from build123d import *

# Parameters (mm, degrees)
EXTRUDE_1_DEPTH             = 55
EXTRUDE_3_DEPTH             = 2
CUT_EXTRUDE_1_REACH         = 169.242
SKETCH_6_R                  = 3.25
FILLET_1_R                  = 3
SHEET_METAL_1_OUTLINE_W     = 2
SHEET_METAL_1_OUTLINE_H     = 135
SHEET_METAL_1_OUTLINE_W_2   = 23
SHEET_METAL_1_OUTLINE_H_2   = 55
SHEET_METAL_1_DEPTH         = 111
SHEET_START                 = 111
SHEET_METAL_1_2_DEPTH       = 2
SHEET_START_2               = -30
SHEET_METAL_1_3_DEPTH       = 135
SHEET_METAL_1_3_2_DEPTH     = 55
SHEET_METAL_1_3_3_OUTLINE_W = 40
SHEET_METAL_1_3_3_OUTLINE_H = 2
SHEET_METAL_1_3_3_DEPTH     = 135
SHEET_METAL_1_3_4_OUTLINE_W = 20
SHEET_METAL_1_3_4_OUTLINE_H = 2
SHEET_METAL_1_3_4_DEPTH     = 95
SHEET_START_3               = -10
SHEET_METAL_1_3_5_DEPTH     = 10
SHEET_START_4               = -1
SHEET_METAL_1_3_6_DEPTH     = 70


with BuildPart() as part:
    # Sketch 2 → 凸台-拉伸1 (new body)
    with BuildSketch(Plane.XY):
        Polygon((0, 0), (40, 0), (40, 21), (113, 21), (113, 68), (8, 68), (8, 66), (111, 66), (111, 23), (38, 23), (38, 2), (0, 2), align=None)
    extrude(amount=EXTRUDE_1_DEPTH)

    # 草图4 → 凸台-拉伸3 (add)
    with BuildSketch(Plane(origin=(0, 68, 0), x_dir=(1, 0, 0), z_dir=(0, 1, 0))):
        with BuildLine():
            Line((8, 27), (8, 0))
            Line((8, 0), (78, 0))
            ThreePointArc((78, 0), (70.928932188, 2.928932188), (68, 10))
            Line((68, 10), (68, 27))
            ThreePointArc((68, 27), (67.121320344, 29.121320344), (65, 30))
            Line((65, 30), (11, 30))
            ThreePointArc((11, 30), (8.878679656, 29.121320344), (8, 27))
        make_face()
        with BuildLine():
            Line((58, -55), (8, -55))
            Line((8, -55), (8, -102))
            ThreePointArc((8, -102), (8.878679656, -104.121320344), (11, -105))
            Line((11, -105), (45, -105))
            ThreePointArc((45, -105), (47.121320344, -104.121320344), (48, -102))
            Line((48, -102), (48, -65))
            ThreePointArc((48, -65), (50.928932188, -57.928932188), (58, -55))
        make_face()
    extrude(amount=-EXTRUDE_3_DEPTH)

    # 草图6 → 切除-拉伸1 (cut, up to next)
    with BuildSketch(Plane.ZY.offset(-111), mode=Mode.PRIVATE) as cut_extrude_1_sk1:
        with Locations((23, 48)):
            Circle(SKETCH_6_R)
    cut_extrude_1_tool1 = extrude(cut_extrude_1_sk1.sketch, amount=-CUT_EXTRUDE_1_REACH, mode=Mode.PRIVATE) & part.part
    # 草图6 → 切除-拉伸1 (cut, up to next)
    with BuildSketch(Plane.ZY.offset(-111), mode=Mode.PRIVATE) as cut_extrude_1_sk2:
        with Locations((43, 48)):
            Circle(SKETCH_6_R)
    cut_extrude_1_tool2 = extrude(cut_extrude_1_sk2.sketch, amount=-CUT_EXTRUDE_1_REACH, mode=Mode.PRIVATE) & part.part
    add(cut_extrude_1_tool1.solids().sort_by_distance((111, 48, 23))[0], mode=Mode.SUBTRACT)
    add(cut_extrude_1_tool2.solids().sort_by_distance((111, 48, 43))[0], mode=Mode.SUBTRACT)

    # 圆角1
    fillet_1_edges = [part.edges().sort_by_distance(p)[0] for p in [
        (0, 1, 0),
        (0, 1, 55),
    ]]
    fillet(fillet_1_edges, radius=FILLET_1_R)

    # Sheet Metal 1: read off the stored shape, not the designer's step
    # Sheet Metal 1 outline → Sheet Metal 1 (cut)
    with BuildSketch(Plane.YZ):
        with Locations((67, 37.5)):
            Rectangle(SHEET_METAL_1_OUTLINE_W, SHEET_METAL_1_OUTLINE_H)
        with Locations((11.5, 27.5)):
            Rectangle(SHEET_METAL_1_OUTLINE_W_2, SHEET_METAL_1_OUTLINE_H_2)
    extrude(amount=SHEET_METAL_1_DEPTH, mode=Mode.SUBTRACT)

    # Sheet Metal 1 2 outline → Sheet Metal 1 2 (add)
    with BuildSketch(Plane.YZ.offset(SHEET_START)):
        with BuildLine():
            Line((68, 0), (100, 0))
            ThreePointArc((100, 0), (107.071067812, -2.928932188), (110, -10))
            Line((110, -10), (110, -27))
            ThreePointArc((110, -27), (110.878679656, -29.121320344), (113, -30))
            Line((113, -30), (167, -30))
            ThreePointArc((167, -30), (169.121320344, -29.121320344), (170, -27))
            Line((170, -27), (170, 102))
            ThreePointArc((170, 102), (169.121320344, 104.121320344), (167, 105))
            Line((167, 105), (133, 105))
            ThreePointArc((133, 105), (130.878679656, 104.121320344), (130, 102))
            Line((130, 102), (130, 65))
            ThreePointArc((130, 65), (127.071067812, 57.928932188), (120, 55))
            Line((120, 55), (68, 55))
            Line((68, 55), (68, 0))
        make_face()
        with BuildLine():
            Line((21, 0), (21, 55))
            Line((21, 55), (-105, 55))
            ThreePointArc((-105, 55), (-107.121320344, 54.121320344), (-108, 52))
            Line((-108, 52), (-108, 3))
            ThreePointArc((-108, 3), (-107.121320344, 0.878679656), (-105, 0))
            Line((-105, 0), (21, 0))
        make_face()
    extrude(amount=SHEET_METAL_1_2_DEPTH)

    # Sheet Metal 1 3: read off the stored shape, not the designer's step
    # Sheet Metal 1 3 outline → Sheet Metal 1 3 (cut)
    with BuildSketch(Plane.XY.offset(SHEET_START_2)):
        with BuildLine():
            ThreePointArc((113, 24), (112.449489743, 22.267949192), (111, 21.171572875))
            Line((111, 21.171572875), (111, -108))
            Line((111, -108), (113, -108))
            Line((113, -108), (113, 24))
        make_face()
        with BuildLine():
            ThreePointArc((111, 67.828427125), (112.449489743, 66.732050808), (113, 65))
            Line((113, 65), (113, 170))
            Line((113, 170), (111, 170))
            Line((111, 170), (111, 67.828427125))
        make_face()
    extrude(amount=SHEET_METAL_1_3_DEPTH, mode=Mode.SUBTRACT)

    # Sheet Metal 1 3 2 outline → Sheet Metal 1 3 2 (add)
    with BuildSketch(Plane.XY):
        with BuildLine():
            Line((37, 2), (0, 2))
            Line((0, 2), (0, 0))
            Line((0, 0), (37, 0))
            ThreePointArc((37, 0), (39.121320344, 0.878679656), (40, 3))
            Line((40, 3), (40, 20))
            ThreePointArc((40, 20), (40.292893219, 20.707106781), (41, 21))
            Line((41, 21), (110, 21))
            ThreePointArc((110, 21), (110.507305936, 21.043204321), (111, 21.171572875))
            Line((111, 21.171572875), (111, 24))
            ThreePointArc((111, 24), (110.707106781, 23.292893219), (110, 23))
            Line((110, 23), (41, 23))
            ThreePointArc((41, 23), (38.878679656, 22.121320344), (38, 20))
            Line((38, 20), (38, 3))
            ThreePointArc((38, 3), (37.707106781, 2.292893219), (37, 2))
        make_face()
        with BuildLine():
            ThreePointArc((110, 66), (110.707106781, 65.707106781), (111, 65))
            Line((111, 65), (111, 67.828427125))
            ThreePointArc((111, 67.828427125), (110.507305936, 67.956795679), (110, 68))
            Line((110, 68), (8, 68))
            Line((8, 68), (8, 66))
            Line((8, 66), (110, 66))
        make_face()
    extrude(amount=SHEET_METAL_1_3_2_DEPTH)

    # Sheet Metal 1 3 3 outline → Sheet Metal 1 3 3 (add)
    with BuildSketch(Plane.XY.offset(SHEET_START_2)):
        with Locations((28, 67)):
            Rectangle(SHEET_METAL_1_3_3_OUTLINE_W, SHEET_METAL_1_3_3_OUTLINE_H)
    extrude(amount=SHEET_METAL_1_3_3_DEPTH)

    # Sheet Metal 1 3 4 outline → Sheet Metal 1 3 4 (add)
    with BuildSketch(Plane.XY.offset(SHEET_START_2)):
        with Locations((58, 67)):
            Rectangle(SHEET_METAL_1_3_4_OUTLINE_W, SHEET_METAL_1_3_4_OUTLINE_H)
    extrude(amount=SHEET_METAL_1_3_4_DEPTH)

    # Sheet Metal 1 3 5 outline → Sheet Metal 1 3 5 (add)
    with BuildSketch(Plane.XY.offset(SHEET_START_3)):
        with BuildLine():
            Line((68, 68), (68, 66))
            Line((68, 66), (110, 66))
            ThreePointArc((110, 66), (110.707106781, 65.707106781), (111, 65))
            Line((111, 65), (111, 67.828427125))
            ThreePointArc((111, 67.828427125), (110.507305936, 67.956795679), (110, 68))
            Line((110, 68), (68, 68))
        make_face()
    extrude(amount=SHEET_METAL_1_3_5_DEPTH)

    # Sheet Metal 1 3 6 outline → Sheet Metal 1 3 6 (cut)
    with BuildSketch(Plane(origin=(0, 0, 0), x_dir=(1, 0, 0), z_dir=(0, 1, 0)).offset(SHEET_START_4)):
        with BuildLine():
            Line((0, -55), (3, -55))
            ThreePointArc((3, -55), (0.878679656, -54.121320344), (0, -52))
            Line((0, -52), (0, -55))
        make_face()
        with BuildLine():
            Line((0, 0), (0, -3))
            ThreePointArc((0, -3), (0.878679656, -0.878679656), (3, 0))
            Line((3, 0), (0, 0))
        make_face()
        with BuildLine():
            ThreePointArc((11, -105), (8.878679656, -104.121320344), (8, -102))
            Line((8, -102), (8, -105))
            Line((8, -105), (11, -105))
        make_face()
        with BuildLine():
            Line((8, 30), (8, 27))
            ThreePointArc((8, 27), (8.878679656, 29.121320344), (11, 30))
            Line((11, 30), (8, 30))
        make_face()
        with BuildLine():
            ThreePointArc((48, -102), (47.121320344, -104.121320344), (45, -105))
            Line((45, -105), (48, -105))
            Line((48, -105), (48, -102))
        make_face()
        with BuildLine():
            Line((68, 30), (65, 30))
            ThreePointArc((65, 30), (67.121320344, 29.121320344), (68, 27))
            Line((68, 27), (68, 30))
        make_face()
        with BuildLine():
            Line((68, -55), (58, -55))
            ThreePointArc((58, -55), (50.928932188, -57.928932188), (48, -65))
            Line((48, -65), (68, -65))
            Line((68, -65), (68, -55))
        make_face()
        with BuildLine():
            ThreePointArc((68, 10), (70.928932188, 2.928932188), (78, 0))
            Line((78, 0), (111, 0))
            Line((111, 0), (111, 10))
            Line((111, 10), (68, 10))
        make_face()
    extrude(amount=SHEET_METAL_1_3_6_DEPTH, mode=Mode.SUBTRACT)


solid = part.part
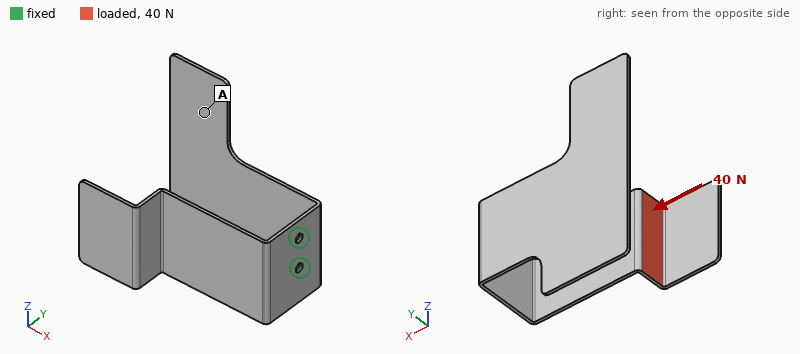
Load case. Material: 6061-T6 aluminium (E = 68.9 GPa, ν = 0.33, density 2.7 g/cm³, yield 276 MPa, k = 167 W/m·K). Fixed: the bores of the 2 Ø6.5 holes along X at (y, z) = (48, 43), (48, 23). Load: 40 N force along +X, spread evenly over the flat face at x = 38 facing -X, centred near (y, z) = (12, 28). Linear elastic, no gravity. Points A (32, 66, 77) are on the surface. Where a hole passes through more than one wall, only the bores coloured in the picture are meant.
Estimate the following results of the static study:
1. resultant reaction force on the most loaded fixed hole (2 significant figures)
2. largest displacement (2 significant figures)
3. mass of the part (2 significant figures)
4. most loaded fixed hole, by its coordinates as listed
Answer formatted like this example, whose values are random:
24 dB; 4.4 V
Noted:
24 N; 1.9 mm; 100 g; (48, 23)
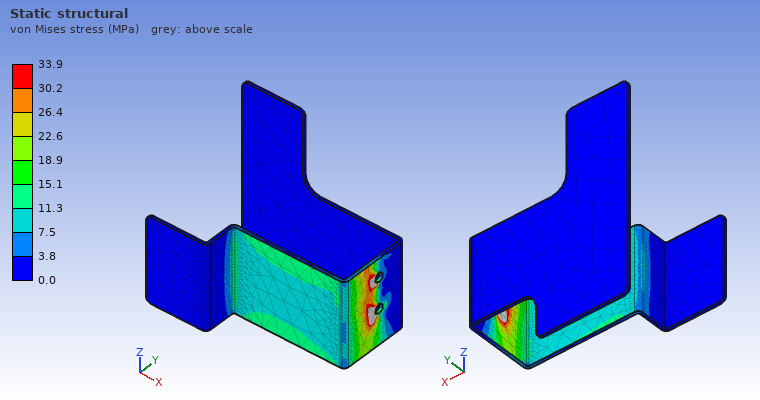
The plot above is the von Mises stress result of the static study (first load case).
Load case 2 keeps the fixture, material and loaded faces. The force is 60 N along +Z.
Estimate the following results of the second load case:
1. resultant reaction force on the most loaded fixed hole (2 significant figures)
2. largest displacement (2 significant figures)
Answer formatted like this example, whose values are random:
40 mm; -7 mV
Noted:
170 N; 1.5 mm
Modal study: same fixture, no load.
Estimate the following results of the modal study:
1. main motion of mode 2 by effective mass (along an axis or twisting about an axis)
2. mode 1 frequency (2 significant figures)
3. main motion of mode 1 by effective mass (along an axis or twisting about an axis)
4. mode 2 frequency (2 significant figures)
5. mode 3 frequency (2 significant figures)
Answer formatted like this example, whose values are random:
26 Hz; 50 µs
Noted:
along Y; 80 Hz; along Y; 86 Hz; 170 Hz
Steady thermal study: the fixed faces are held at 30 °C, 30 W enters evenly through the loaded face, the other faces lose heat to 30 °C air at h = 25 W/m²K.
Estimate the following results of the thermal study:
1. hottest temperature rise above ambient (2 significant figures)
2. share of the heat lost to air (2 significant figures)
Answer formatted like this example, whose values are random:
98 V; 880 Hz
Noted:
79 K; 66 %
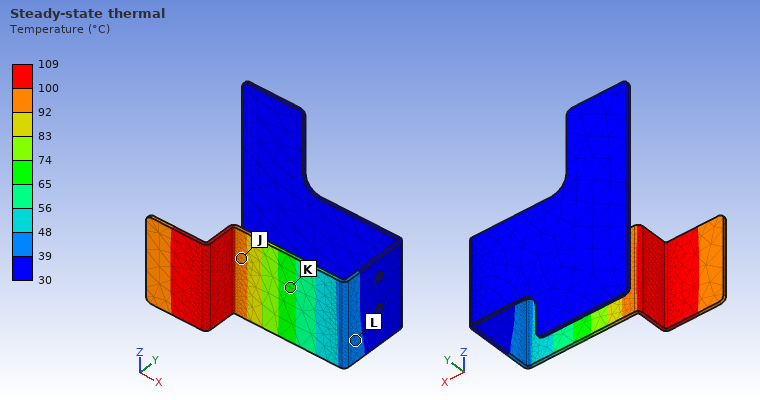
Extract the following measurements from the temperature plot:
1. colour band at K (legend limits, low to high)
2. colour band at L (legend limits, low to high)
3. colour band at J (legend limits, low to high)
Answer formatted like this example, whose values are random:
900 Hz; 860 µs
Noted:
65 to 74 °C; 39 to 48 °C; 92 to 100 °C
